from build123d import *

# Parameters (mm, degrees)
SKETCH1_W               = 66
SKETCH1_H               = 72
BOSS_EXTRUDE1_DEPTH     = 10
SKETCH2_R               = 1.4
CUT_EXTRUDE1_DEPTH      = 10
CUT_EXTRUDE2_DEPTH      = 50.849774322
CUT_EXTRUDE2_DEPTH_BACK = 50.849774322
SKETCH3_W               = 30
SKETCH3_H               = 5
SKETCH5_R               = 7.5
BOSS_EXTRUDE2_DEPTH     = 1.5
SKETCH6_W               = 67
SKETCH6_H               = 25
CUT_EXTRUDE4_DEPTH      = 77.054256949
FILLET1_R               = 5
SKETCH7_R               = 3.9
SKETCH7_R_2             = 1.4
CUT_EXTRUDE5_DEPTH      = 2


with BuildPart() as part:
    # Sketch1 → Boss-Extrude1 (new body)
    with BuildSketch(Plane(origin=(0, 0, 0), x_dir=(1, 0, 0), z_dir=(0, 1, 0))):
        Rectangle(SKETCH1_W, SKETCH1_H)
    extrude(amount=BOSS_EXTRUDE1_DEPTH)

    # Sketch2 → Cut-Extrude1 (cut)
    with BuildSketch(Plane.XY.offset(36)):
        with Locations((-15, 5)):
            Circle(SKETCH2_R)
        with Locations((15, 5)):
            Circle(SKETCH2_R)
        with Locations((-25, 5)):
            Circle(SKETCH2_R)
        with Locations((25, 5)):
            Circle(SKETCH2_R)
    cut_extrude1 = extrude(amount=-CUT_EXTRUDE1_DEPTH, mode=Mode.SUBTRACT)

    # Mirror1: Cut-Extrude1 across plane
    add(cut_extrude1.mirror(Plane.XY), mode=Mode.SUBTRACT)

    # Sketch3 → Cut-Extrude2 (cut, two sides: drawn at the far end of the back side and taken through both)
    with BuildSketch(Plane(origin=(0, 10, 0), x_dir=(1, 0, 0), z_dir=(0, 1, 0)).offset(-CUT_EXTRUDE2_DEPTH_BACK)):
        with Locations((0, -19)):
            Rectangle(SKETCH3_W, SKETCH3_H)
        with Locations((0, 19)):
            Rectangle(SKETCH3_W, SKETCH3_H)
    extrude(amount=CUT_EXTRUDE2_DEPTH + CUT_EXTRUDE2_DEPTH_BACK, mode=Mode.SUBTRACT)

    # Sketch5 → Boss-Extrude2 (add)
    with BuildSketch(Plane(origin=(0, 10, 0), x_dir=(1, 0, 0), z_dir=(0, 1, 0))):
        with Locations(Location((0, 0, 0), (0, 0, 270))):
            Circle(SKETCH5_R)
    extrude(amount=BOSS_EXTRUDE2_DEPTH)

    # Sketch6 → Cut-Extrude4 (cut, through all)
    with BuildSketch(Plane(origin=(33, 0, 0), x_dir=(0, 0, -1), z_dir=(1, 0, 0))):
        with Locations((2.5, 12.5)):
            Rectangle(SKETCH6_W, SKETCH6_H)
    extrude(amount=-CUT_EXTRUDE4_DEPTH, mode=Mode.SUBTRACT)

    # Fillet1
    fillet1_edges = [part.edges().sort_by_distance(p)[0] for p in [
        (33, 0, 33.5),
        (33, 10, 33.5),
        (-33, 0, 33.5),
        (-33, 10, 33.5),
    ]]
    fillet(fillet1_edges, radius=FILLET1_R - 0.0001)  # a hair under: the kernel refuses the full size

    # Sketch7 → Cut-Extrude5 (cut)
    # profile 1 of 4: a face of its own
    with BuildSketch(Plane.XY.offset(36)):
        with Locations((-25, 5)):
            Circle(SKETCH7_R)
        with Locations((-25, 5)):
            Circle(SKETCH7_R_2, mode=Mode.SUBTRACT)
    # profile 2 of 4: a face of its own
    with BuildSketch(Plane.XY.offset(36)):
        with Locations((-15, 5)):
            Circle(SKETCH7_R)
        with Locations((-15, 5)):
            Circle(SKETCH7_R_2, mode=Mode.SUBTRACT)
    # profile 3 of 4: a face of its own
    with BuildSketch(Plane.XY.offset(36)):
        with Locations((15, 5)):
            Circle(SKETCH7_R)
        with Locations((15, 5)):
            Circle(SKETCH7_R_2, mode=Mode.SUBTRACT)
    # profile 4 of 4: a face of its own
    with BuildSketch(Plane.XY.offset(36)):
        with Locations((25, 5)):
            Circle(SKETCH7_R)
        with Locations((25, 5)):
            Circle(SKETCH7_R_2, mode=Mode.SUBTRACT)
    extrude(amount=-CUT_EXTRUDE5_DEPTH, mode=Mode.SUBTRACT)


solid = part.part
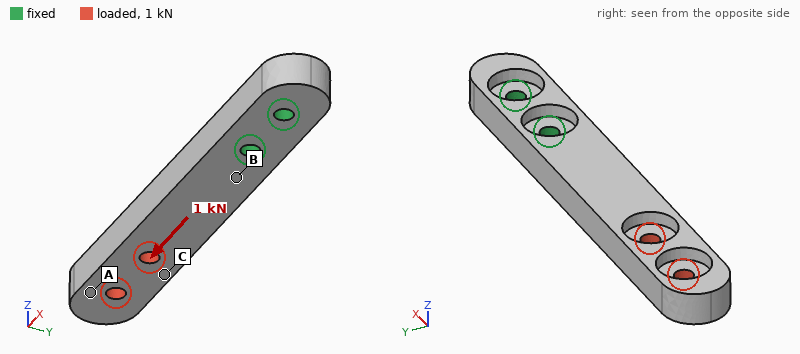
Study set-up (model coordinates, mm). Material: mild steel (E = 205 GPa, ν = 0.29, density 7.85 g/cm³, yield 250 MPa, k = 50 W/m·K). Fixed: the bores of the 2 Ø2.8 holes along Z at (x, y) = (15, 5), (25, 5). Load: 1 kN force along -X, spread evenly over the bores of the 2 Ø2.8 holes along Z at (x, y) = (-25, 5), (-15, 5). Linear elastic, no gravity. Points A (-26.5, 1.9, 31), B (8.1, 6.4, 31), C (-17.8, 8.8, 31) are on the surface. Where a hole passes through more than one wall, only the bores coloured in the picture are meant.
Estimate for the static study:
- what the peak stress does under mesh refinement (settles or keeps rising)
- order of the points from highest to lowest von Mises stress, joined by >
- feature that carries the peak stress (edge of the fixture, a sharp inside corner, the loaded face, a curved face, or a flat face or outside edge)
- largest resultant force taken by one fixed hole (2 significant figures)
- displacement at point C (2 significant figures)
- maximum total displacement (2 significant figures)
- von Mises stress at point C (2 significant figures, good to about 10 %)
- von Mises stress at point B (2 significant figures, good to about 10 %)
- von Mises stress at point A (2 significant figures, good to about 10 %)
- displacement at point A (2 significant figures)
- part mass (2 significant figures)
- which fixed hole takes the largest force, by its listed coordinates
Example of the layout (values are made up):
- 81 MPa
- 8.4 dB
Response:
- keeps rising
- B > C > A
- edge of the fixture
- 860 N
- 23 µm
- 44 µm
- 33 MPa
- 46 MPa
- 11 MPa
- 35 µm
- 21 g
- (15, 5)
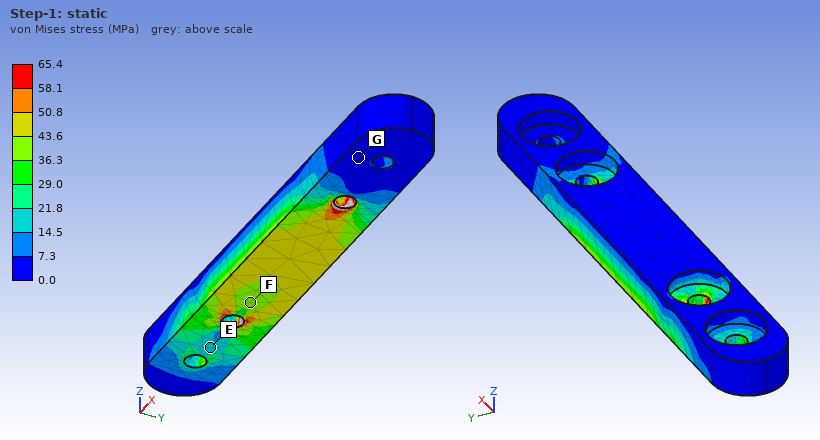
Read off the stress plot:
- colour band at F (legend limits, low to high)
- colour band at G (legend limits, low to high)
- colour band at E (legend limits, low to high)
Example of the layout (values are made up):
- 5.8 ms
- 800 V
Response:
- 36.3 to 43.6 MPa
- 0.0 to 7.3 MPa
- 14.5 to 21.8 MPa
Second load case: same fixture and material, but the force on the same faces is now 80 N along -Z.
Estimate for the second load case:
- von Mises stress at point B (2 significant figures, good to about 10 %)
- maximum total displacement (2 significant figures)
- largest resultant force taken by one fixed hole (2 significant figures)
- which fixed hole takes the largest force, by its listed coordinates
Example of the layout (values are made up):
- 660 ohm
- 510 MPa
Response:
- 55 MPa
- 0.12 mm
- 240 N
- (15, 5)
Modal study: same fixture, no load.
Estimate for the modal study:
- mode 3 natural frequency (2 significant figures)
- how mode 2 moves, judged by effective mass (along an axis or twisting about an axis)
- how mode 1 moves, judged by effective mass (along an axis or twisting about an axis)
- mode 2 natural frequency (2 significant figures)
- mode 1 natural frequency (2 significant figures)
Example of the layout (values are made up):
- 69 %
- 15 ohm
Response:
- 9000 Hz
- along Y
- along Z
- 3300 Hz
- 1700 Hz
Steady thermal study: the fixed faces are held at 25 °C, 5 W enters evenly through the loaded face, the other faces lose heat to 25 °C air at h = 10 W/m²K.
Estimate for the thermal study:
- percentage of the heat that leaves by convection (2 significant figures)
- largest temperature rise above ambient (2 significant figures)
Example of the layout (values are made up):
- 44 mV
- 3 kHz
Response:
- 14 %
- 76 K
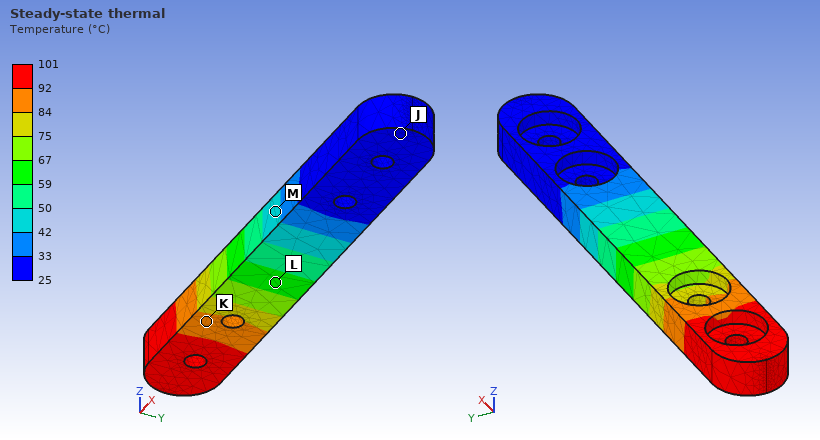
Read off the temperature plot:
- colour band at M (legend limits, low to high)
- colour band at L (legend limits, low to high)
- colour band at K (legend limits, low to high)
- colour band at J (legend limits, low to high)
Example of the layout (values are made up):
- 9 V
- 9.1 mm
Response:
- 42 to 50 °C
- 59 to 67 °C
- 84 to 92 °C
- 25 to 33 °C
